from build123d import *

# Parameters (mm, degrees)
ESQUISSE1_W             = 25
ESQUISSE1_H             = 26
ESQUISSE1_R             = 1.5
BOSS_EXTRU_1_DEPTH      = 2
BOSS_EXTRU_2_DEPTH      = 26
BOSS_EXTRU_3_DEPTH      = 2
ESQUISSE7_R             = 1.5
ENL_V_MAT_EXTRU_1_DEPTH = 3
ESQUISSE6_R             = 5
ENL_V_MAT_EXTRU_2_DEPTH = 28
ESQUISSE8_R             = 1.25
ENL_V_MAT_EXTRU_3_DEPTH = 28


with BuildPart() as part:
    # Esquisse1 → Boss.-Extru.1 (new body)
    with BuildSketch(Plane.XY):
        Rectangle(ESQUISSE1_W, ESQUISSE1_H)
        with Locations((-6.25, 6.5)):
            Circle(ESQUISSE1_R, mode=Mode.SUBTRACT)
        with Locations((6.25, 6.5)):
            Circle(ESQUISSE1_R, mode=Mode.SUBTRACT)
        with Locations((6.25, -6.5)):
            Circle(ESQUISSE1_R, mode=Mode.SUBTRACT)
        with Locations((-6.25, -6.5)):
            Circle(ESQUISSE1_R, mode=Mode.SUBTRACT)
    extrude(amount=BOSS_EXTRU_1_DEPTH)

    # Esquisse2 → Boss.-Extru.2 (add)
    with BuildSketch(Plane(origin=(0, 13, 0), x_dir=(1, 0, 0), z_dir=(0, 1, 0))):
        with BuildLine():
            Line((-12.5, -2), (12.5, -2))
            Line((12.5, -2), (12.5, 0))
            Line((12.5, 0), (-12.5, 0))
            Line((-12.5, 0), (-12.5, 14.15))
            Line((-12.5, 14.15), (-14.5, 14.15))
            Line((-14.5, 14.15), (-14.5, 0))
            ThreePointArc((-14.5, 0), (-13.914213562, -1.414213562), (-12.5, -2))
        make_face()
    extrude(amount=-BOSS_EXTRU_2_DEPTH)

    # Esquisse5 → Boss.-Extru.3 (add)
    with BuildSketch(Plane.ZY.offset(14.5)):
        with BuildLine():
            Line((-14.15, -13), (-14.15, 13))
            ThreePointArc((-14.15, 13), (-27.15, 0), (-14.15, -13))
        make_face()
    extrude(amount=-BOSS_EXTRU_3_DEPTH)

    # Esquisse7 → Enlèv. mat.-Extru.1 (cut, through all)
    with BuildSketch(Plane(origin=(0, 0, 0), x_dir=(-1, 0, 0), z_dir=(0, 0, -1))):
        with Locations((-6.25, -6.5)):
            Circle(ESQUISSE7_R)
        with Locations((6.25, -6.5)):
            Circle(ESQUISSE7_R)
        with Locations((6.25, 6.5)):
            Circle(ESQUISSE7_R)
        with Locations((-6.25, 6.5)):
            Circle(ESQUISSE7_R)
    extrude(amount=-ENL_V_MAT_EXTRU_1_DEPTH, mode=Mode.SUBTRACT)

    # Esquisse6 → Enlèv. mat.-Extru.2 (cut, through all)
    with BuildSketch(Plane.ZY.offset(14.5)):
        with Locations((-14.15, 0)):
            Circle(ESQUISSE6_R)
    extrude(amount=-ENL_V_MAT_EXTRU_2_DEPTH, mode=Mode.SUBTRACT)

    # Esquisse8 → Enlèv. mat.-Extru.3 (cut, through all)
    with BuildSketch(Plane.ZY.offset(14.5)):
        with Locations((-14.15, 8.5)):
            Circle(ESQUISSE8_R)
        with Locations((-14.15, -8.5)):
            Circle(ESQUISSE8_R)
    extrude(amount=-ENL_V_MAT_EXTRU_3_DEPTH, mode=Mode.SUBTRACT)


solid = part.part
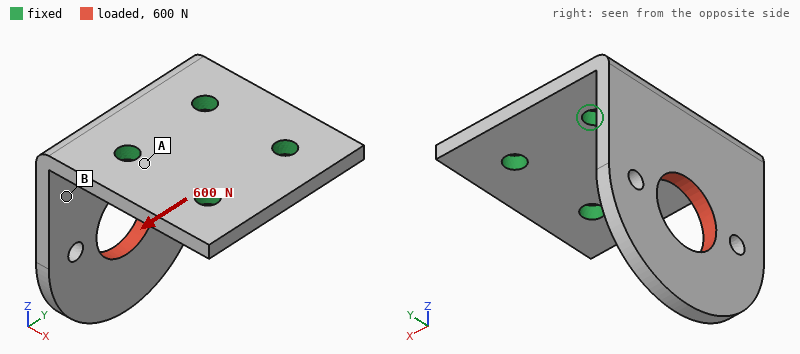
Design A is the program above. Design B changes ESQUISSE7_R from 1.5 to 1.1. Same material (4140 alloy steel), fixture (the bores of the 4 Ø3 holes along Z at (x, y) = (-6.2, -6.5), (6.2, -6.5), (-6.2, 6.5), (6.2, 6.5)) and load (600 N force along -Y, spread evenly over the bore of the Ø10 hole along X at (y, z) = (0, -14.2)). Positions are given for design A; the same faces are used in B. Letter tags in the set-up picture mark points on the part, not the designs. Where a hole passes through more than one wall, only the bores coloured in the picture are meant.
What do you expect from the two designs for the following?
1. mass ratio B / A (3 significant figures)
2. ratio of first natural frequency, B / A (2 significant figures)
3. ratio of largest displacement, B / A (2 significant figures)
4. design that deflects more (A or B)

1.01
0.98
1.2
B
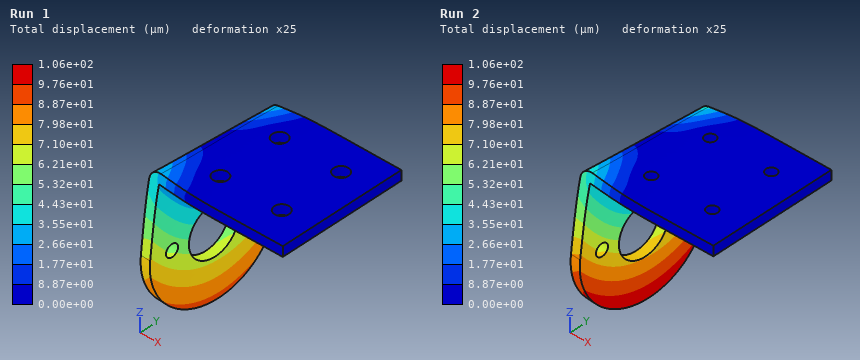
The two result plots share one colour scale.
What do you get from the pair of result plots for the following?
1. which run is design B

Run 2
